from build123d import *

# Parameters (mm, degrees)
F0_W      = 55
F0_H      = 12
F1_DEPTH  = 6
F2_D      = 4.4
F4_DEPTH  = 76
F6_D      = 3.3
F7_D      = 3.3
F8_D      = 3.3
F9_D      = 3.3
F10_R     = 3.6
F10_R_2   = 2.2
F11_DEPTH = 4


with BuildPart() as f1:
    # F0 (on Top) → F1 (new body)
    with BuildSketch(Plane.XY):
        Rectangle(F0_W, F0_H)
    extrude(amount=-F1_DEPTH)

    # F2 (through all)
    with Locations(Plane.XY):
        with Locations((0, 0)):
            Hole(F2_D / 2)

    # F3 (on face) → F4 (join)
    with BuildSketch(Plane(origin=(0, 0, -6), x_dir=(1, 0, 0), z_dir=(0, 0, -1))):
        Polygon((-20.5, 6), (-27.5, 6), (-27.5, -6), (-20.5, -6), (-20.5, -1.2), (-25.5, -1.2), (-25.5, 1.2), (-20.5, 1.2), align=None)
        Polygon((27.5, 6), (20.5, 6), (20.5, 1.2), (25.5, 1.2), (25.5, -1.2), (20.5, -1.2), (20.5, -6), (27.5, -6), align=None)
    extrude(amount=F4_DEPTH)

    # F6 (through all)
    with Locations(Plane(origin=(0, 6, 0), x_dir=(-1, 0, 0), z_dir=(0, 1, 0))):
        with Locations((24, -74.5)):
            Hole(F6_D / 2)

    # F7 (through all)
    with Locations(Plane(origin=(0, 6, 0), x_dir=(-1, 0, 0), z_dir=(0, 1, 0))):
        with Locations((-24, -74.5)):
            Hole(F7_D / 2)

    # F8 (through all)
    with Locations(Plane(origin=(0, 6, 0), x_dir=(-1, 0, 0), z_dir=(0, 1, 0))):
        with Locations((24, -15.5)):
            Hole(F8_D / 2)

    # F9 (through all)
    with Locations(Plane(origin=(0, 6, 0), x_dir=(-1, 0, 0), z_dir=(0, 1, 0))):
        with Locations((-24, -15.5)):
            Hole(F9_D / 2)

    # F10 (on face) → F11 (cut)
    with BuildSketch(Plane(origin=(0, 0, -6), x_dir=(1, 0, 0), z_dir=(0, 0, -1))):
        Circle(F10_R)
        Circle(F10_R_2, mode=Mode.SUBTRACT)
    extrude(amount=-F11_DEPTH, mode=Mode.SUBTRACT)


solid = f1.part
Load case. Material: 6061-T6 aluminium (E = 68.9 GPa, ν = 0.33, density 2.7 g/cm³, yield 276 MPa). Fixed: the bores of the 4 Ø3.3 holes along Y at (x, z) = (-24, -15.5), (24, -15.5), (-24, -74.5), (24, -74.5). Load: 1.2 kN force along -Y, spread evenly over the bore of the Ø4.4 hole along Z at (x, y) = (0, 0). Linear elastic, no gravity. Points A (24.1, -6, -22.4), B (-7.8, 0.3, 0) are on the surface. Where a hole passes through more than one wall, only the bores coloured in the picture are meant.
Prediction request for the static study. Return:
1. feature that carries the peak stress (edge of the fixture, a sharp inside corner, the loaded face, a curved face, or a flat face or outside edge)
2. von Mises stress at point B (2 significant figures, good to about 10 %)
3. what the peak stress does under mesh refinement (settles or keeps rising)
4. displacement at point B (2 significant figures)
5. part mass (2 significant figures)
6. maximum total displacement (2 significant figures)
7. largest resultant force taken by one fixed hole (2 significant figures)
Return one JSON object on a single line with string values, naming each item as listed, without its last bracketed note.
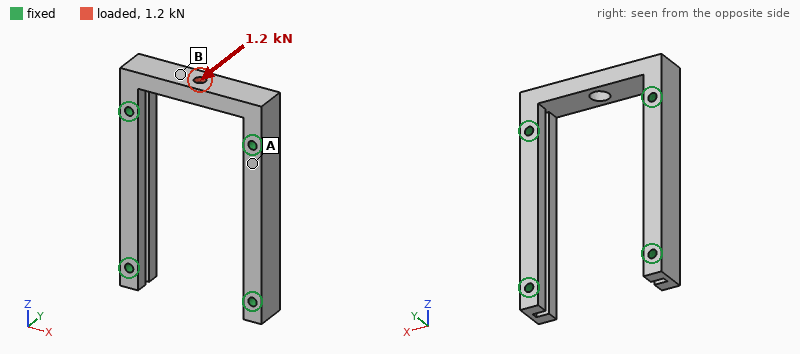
{"feature that carries the peak stress": "edge of the fixture", "von Mises stress at point B": "37 MPa", "what the peak stress does under mesh refinement": "keeps rising", "displacement at point B": "50 µm", "part mass": "39 g", "maximum total displacement": "61 µm", "largest resultant force taken by one fixed hole": "600 N"}
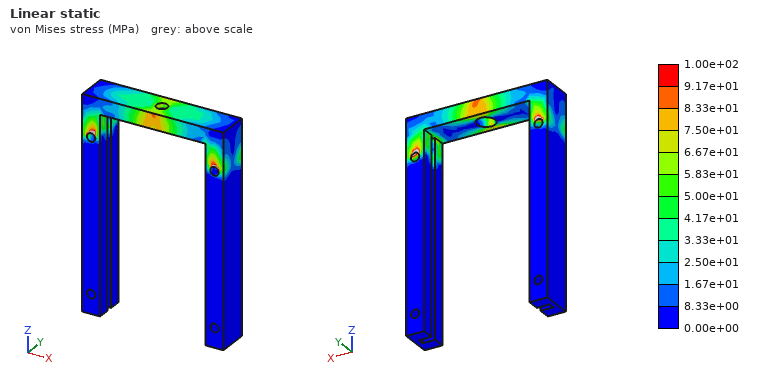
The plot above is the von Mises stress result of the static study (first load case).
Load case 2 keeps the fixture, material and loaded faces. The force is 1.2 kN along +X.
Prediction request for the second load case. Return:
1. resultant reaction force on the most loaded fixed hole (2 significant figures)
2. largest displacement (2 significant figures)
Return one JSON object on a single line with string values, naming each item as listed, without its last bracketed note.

{"resultant reaction force on the most loaded fixed hole": "630 N", "largest displacement": "18 µm"}
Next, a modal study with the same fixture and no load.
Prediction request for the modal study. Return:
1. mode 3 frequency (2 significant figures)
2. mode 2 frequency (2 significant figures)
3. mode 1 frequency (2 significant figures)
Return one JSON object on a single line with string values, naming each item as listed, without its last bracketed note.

{"mode 3 frequency": "11 kHz", "mode 2 frequency": "9400 Hz", "mode 1 frequency": "9300 Hz"}
